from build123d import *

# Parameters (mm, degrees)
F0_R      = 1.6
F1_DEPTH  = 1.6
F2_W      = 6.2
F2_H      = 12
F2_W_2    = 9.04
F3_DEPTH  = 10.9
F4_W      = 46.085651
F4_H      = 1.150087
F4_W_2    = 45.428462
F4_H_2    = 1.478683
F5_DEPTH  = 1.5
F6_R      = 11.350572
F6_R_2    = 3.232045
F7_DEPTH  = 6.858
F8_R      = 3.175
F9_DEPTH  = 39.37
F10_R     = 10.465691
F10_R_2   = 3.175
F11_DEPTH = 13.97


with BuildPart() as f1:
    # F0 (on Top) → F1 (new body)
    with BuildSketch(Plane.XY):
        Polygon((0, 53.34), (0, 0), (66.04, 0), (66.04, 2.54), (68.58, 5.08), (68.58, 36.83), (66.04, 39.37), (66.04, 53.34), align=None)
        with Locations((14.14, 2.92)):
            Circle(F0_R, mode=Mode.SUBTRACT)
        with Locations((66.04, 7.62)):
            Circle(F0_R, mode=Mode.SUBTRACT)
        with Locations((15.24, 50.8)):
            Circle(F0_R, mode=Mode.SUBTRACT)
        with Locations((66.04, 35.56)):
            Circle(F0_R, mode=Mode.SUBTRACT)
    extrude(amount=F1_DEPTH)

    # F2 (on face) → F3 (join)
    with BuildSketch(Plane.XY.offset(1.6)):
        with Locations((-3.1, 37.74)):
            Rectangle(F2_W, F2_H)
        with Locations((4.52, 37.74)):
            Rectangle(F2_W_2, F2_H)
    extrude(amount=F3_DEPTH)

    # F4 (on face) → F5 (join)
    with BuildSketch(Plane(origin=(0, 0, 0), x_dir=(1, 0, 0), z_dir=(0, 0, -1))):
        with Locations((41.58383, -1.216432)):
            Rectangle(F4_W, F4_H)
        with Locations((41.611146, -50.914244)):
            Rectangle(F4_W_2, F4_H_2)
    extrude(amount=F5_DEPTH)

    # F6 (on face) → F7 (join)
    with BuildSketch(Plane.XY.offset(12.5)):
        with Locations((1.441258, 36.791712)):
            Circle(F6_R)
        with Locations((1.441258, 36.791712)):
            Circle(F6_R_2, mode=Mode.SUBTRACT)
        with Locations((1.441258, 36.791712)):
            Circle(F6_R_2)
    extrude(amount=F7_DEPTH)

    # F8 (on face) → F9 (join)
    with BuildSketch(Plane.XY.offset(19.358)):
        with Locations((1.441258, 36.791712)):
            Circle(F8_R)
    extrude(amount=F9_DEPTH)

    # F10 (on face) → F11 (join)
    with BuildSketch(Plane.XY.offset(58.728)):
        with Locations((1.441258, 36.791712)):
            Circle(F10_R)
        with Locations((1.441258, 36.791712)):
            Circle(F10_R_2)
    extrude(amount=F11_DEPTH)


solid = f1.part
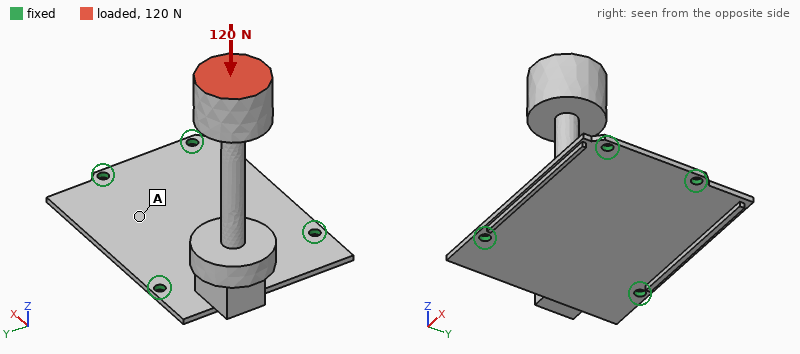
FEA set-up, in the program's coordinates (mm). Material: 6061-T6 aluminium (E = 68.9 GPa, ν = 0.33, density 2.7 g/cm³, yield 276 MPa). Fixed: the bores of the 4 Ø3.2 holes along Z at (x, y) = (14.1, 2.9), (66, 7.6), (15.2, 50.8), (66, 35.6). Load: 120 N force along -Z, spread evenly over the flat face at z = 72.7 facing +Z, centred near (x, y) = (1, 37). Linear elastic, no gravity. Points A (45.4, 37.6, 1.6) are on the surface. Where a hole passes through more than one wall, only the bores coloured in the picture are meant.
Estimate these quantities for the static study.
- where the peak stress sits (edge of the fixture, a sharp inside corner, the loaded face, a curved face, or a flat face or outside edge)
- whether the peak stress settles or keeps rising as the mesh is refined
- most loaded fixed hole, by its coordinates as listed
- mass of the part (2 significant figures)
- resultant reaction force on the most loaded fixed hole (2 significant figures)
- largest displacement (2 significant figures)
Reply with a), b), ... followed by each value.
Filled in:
a) edge of the fixture
b) keeps rising
c) (15.2, 50.8)
d) 45 g
e) 94 N
f) 1.2 mm
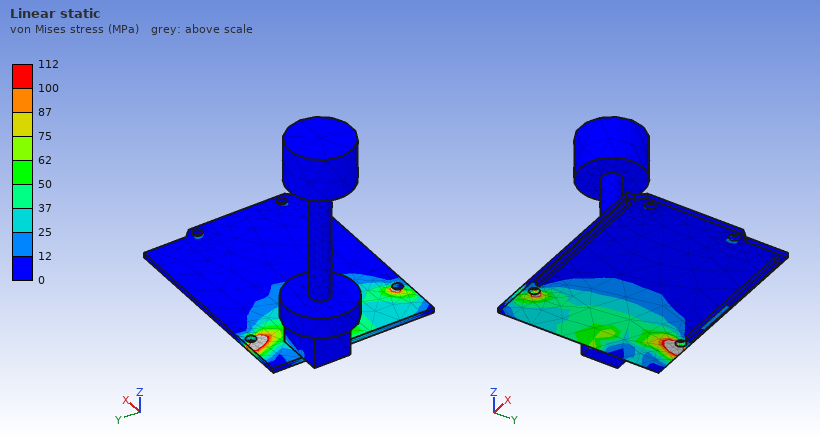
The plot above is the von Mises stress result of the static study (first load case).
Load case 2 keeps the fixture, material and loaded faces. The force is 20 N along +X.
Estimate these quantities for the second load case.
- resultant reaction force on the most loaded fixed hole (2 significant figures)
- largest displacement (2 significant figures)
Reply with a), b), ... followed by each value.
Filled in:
a) 12 N
b) 1.4 mm
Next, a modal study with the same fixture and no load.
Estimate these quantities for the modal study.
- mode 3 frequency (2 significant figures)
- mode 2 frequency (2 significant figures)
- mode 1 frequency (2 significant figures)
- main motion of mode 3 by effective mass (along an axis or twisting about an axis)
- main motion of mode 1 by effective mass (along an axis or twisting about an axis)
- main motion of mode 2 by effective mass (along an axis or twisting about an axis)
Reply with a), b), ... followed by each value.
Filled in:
a) 1200 Hz
b) 270 Hz
c) 170 Hz
d) along Z
e) along X
f) along Y
